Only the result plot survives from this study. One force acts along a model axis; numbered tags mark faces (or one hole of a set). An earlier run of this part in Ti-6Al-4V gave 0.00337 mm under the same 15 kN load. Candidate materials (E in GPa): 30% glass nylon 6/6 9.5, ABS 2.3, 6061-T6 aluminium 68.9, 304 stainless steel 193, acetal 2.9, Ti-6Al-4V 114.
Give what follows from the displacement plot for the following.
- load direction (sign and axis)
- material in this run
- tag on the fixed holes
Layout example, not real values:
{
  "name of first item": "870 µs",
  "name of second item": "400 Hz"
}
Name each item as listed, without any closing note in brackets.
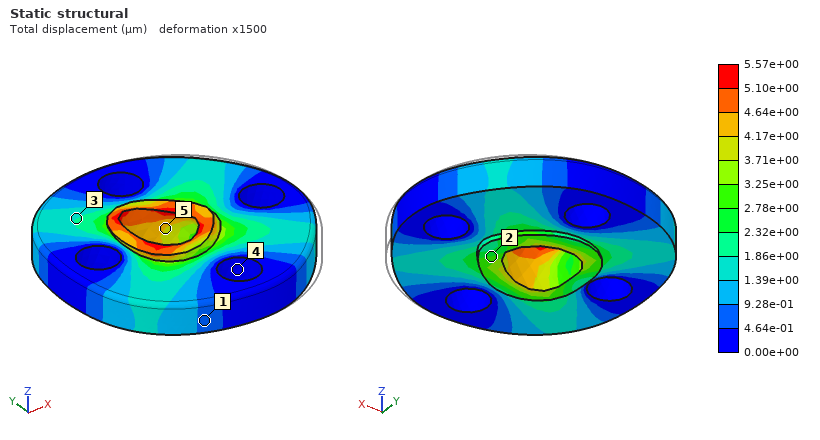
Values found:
{
  "load direction": "-X",
  "material in this run": "6061-T6 aluminium",
  "tag on the fixed holes": "4"
}
